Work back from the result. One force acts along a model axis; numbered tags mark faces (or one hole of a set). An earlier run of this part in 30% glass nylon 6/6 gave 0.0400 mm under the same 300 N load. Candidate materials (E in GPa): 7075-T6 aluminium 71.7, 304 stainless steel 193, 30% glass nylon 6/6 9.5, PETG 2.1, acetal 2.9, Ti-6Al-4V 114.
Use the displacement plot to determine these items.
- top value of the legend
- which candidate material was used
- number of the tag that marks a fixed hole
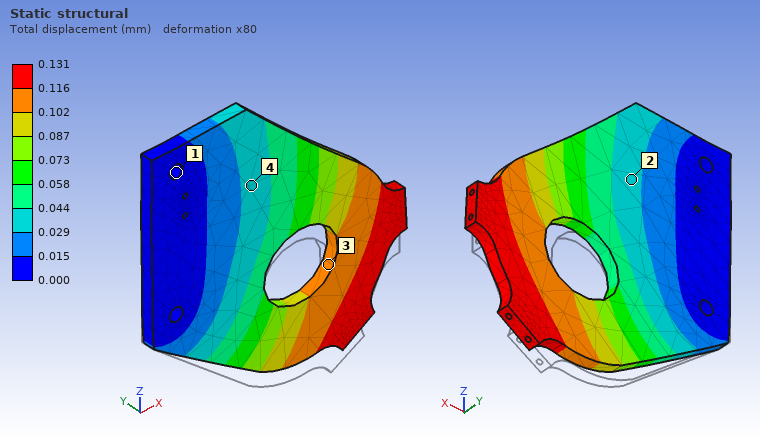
0.131 mm
acetal
1
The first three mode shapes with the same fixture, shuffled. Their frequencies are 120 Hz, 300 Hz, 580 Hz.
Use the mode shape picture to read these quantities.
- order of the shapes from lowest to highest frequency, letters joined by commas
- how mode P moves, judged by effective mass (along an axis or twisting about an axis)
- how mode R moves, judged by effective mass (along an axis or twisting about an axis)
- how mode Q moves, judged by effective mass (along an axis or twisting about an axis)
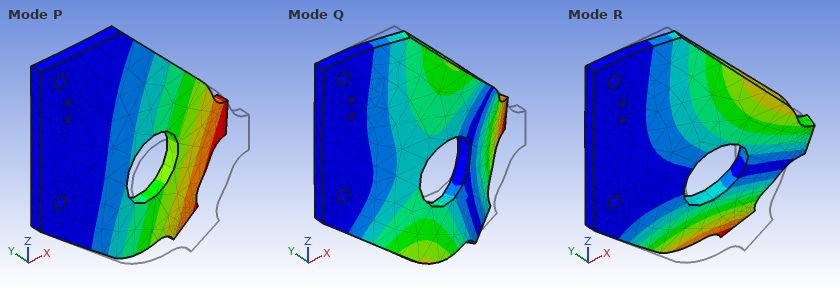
P, R, Q
along Y
twisting about X
along Y
